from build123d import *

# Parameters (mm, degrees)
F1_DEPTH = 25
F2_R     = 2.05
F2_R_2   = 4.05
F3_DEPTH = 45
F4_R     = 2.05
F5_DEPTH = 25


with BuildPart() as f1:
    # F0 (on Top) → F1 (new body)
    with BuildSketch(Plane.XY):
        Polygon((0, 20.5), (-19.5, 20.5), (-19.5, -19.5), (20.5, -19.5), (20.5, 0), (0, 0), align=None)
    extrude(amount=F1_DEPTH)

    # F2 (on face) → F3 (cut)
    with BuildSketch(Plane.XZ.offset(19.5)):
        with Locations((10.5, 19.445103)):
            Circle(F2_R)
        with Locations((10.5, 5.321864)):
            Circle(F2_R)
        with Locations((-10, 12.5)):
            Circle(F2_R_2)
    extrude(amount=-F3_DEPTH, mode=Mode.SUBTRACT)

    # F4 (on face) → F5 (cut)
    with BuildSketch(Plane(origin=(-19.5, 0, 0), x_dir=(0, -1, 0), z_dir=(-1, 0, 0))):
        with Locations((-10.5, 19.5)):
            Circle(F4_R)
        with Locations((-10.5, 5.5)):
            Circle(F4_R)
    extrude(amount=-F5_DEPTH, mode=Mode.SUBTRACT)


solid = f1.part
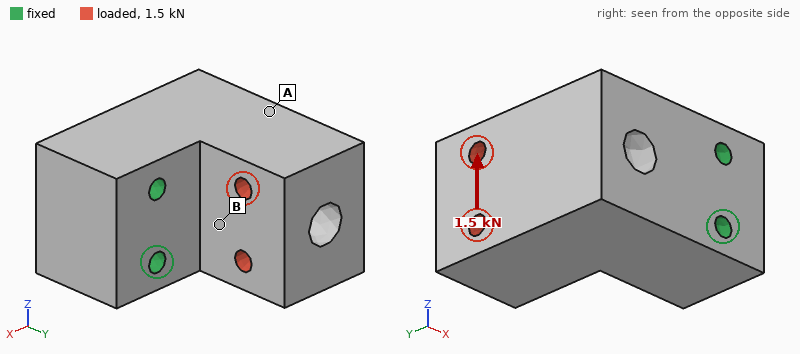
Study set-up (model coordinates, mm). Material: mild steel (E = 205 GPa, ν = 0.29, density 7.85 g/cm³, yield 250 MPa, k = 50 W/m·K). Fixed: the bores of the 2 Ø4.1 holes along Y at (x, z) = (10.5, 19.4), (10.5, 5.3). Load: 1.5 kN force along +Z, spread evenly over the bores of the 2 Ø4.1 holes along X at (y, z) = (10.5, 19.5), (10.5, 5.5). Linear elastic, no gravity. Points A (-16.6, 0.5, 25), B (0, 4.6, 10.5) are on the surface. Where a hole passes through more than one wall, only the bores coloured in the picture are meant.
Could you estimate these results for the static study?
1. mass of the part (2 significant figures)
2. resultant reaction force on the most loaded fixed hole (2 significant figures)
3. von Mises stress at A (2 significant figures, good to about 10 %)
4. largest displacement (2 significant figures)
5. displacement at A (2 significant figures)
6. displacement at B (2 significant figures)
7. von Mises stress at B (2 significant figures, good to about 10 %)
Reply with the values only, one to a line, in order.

210 g
2.2 kN
4.2 MPa
8.7 µm
4.7 µm
3.5 µm
13 MPa
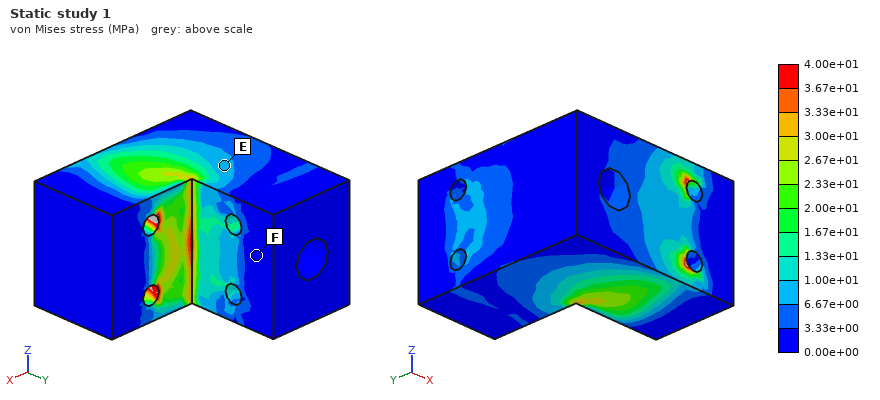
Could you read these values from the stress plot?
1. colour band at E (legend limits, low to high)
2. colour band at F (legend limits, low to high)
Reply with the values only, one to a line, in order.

6.67e+00 to 1.00e+01 MPa
0.00e+00 to 3.33e+00 MPa
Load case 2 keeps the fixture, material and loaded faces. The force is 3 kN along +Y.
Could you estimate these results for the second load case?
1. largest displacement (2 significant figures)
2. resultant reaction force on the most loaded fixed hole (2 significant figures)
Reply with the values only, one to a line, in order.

10 µm
1.5 kN
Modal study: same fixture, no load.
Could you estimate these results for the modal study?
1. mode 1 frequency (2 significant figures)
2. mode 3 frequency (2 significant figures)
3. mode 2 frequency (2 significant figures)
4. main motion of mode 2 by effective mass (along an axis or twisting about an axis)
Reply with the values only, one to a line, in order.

7900 Hz
15 kHz
8900 Hz
along Z
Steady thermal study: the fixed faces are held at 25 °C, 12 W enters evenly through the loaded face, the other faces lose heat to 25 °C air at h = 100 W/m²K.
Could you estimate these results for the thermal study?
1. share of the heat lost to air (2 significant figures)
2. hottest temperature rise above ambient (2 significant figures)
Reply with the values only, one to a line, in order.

35 %
13 K
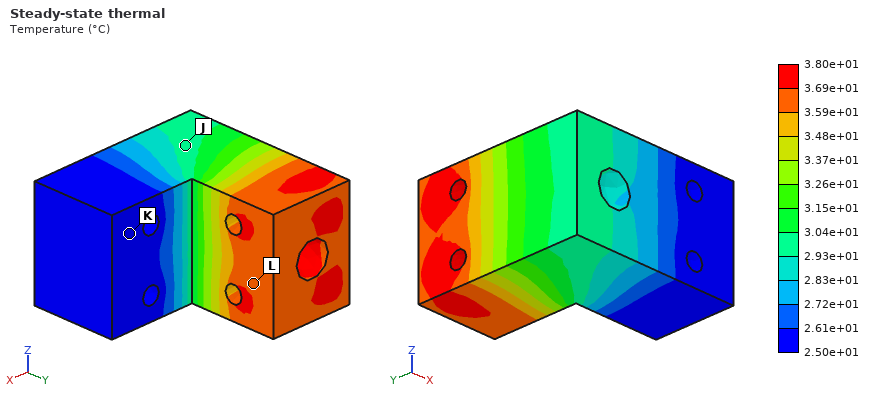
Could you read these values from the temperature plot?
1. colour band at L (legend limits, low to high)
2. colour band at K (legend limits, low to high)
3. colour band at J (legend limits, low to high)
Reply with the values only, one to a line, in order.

3.59e+01 to 3.69e+01 °C
2.50e+01 to 2.61e+01 °C
2.93e+01 to 3.04e+01 °C
